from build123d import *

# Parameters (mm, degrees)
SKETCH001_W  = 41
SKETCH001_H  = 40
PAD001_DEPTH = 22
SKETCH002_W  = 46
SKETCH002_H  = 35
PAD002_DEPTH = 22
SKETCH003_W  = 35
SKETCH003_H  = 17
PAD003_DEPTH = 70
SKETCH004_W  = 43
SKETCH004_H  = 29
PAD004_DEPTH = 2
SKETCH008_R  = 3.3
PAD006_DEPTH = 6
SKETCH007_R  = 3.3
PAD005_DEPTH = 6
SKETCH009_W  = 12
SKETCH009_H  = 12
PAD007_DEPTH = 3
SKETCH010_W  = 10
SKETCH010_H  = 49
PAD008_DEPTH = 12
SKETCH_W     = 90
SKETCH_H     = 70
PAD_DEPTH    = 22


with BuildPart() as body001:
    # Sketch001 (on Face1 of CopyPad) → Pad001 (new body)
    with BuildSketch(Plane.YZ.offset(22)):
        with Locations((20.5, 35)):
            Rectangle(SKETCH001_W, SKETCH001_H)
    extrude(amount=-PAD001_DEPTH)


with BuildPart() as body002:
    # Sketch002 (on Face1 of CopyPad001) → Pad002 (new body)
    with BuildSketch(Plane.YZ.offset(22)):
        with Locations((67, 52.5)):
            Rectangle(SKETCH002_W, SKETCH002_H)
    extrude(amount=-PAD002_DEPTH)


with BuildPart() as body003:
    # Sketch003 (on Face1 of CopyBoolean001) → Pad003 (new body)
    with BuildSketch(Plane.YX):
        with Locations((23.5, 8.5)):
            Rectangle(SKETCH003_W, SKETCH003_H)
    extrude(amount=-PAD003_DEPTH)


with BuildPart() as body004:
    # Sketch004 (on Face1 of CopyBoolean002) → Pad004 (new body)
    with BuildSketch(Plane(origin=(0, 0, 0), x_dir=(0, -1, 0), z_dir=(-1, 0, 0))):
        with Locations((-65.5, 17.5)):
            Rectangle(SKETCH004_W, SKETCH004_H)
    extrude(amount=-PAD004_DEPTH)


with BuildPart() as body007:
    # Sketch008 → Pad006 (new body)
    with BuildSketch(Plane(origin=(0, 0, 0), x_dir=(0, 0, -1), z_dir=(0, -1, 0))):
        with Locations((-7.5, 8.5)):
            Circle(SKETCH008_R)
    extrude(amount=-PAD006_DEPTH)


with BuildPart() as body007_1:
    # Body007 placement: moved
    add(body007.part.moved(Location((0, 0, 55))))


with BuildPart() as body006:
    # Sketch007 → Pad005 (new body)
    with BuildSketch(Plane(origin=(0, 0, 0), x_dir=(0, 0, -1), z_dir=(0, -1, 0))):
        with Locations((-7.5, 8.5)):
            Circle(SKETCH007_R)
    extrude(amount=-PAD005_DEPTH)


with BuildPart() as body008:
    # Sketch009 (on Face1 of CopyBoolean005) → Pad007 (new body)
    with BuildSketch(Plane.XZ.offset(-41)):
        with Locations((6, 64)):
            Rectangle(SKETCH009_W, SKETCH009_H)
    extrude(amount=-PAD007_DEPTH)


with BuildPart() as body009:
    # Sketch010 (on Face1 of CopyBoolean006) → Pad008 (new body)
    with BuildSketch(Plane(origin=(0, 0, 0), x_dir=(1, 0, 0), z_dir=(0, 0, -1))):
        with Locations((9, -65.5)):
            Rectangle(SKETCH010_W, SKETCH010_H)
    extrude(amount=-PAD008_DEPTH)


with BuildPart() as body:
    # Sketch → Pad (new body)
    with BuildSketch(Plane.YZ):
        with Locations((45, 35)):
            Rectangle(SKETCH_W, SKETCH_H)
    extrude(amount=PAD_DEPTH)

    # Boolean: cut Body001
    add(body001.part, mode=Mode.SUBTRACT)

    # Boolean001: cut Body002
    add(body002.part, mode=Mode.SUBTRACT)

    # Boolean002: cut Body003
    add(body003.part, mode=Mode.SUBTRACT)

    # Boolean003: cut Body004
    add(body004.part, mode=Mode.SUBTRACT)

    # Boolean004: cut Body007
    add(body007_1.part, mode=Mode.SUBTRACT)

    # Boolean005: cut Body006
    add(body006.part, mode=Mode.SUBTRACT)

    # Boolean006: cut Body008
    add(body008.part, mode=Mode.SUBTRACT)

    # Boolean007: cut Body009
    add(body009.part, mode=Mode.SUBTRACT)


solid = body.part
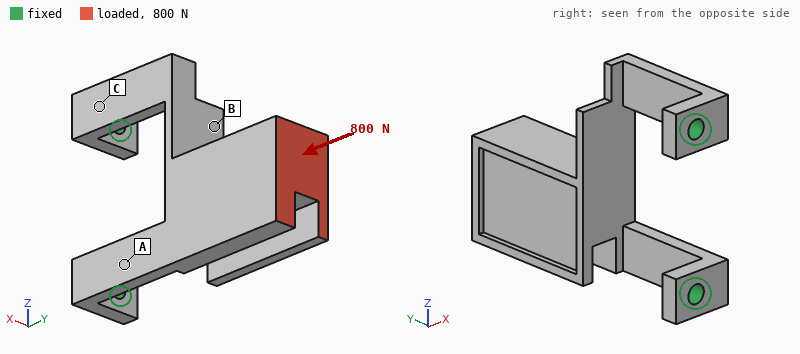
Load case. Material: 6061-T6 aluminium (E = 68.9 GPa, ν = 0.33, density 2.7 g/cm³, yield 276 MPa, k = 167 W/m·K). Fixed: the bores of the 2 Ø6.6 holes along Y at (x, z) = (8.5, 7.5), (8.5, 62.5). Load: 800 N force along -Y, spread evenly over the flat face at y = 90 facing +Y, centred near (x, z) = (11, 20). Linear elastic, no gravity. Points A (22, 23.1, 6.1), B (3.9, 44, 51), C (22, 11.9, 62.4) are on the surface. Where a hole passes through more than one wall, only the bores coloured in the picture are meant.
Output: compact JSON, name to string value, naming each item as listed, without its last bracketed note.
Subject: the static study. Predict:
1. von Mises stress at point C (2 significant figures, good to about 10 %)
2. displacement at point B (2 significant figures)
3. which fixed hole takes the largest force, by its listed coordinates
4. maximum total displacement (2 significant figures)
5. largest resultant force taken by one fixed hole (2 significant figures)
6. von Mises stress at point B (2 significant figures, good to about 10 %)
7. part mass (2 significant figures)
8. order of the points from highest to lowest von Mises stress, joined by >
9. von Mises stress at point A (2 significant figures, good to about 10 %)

{"von Mises stress at point C": "35 MPa", "displacement at point B": "0.32 mm", "which fixed hole takes the largest force, by its listed coordinates": "(8.5, 7.5)", "maximum total displacement": "1.1 mm", "largest resultant force taken by one fixed hole": "650 N", "von Mises stress at point B": "13 MPa", "part mass": "110 g", "order of the points from highest to lowest von Mises stress, joined by >": "A > C > B", "von Mises stress at point A": "63 MPa"}
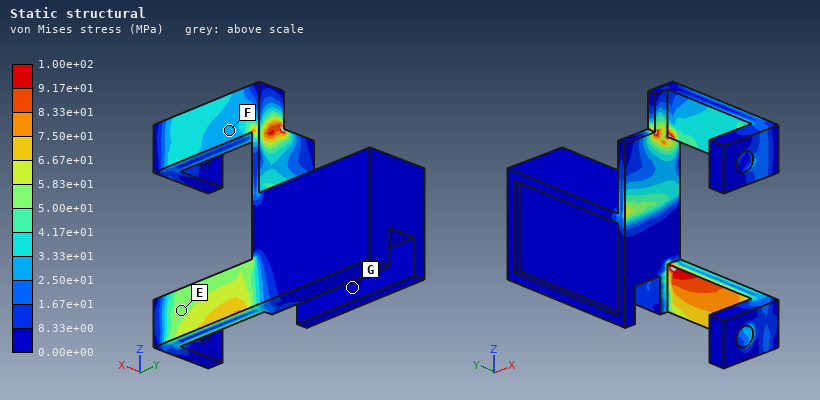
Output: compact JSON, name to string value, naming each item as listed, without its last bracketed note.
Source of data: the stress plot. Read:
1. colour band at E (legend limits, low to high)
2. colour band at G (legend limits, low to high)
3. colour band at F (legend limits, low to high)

{"colour band at E": "5.00e+01 to 5.83e+01 MPa", "colour band at G": "0.00e+00 to 8.33e+00 MPa", "colour band at F": "2.50e+01 to 3.33e+01 MPa"}
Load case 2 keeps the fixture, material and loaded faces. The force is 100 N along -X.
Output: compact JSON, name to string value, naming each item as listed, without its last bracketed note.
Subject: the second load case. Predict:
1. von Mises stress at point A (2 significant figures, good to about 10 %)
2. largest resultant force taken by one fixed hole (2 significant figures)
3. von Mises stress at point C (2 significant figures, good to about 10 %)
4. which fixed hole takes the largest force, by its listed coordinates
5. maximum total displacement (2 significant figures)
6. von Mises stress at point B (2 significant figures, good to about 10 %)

{"von Mises stress at point A": "70 MPa", "largest resultant force taken by one fixed hole": "58 N", "von Mises stress at point C": "48 MPa", "which fixed hole takes the largest force, by its listed coordinates": "(8.5, 62.5)", "maximum total displacement": "1.3 mm", "von Mises stress at point B": "16 MPa"}
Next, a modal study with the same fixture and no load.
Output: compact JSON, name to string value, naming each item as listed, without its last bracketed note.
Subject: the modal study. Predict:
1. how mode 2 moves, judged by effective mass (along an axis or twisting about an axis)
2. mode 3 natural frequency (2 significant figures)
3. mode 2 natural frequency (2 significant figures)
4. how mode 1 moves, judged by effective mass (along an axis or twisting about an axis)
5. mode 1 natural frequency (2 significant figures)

{"how mode 2 moves, judged by effective mass": "along Z", "mode 3 natural frequency": "1500 Hz", "mode 2 natural frequency": "810 Hz", "how mode 1 moves, judged by effective mass": "along X", "mode 1 natural frequency": "230 Hz"}
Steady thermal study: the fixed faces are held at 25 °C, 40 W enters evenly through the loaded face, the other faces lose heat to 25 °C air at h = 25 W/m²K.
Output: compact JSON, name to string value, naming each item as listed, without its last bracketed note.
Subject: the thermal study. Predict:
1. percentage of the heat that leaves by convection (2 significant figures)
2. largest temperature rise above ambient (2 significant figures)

{"percentage of the heat that leaves by convection": "41 %", "largest temperature rise above ambient": "78 K"}
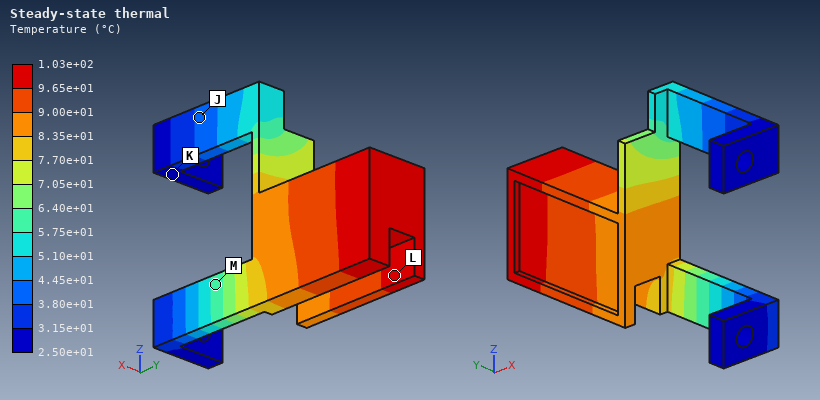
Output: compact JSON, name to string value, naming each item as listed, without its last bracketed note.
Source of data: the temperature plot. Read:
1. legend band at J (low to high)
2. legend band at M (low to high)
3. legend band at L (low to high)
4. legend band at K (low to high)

{"legend band at J": "3.80e+01 to 4.45e+01 °C", "legend band at M": "5.75e+01 to 6.40e+01 °C", "legend band at L": "9.65e+01 to 1.03e+02 °C", "legend band at K": "2.50e+01 to 3.15e+01 °C"}
